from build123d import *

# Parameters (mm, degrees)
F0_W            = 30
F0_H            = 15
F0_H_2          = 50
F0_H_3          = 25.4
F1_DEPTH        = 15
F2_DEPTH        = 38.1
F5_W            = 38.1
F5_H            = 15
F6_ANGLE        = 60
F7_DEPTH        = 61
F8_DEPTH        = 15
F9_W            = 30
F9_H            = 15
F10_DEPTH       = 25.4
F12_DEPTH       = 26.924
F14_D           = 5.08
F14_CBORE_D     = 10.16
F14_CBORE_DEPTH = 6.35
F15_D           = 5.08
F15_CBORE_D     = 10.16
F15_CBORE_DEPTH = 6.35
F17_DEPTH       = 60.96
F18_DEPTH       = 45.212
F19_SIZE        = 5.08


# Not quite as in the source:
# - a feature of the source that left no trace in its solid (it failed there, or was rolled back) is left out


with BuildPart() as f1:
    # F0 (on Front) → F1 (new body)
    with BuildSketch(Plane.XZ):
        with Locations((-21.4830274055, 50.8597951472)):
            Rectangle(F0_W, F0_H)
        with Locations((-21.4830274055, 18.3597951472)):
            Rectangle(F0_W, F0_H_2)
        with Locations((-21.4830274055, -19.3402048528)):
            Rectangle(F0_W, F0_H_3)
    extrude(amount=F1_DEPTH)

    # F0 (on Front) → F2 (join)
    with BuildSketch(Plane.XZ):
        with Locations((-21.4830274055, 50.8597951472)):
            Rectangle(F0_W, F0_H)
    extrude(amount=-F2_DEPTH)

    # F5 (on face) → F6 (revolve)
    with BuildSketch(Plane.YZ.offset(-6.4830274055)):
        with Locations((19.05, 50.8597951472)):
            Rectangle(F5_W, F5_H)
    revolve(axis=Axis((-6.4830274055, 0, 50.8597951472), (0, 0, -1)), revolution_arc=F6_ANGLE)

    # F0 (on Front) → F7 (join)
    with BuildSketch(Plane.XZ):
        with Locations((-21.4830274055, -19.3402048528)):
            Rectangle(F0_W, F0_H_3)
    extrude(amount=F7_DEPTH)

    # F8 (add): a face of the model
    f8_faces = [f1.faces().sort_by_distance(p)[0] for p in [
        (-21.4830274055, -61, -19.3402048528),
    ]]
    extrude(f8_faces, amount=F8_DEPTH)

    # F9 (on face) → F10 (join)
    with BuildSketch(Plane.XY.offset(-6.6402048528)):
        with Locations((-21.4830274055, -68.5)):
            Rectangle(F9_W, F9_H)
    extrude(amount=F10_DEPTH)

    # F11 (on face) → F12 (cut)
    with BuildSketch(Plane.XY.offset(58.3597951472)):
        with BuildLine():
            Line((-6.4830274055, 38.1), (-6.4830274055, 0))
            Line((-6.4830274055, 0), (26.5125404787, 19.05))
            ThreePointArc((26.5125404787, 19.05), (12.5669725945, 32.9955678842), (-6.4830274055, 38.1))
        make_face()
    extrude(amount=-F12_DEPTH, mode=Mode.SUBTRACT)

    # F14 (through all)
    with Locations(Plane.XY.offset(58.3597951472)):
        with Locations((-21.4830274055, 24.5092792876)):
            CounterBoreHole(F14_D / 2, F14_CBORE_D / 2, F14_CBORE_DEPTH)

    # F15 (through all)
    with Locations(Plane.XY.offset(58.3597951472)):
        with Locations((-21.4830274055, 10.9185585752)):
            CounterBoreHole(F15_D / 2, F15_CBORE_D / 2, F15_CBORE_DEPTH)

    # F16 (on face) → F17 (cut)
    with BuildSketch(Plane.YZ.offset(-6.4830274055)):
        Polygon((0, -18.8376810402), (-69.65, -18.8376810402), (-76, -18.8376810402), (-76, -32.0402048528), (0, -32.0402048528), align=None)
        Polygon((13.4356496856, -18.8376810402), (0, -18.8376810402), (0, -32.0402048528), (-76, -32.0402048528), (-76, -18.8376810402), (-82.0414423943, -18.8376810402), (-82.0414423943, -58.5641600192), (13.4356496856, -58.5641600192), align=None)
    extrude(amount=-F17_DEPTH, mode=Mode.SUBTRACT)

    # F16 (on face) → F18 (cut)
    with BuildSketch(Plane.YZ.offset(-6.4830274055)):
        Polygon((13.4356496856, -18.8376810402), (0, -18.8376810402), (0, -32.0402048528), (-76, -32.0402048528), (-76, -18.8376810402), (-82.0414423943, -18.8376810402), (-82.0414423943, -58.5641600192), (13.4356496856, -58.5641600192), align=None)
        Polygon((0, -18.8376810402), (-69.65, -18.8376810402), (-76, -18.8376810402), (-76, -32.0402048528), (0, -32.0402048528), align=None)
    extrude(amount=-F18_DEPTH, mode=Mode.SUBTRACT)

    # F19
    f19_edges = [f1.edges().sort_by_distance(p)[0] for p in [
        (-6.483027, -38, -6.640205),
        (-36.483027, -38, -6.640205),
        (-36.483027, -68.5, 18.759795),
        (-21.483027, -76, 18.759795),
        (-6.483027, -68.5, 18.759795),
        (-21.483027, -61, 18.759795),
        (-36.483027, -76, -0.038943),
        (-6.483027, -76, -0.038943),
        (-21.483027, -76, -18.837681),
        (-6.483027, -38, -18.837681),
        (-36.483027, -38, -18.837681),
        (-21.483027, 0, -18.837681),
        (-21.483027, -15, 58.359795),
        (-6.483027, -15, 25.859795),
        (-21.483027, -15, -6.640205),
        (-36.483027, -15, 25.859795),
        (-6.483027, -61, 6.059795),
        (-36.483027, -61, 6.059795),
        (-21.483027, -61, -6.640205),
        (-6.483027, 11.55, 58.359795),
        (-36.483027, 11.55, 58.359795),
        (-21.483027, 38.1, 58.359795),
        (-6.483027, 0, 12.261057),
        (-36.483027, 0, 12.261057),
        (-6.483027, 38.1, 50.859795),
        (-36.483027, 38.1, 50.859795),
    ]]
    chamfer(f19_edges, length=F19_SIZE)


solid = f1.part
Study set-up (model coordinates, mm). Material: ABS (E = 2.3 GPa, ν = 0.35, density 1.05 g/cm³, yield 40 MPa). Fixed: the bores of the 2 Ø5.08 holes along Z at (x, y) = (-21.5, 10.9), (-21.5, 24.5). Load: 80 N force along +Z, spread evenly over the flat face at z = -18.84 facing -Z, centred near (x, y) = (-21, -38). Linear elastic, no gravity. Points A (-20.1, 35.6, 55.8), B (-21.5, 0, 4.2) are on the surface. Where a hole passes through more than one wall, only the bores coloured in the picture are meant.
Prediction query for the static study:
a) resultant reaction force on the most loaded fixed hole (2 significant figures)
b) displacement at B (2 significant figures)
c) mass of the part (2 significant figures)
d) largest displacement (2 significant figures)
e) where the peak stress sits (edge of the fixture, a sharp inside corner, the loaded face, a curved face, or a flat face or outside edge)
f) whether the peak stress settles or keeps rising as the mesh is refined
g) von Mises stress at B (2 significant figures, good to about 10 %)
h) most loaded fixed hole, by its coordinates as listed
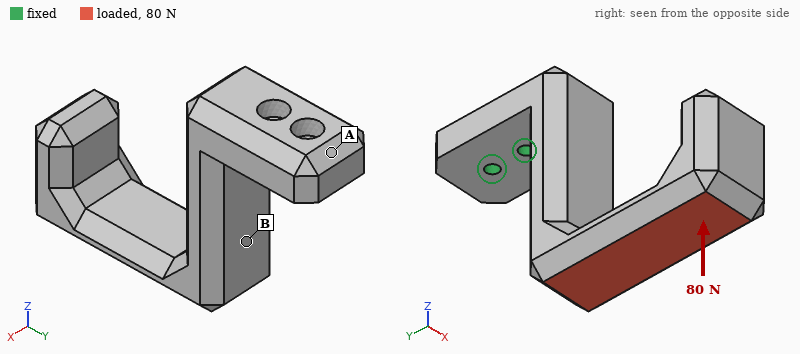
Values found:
230 N
0.39 mm
77 g
1.4 mm
edge of the fixture
keeps rising
2.2 MPa
(-21.5, 10.9)
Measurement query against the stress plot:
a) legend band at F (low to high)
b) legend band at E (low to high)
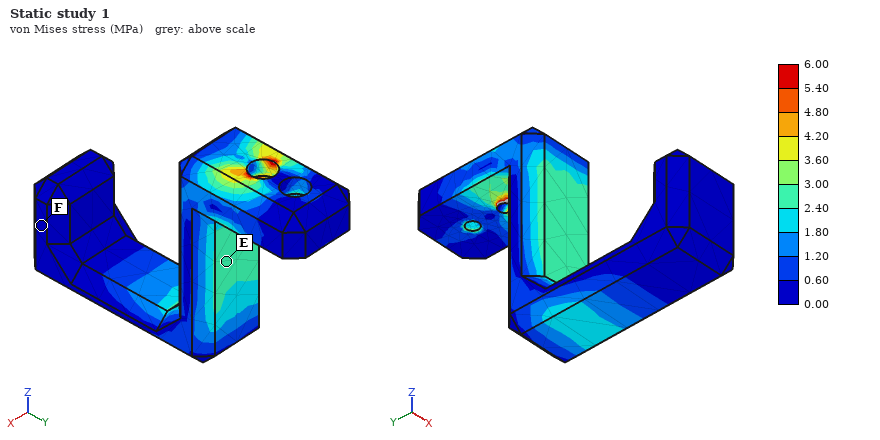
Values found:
0.00 to 0.60 MPa
2.40 to 3.00 MPa
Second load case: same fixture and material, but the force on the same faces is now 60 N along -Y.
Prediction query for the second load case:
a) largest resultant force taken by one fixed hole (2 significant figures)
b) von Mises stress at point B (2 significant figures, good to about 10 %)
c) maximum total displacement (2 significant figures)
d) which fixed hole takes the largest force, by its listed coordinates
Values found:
200 N
1.5 MPa
1.4 mm
(-21.5, 10.9)
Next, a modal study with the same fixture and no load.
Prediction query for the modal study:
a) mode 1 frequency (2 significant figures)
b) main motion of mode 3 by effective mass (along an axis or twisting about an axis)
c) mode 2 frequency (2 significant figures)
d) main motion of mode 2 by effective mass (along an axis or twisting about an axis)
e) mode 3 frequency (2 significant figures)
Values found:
170 Hz
along Y
230 Hz
along X
470 Hz
